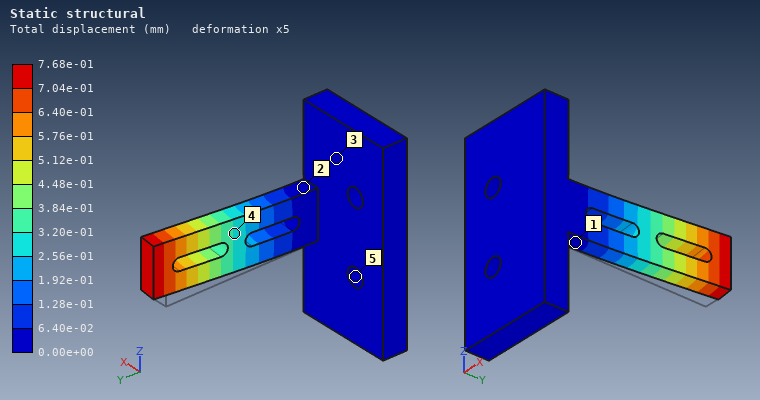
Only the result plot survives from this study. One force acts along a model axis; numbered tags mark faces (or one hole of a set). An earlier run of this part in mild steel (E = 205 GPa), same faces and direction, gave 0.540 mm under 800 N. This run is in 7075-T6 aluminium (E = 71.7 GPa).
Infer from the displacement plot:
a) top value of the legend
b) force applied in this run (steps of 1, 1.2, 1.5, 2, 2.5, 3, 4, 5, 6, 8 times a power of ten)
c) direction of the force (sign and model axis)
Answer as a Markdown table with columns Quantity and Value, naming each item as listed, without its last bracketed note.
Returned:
| Quantity | Value |
|---|---|
| top value of the legend | 7.68e-01 mm |
| force applied in this run | 400 N |
| direction of the force | +X |
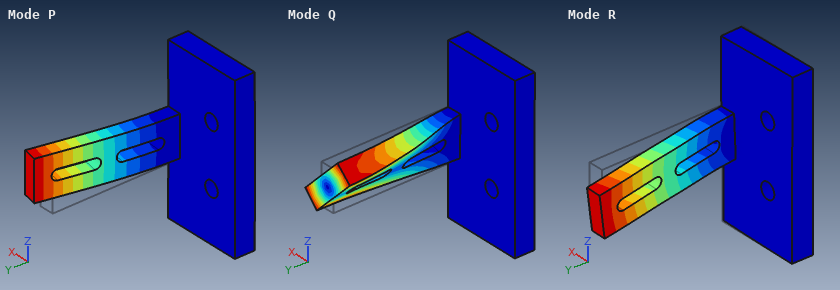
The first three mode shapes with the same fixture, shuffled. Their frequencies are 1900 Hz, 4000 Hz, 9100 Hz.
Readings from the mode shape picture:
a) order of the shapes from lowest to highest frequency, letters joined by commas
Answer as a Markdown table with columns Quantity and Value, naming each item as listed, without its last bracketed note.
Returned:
| Quantity | Value |
|---|---|
| order of the shapes from lowest to highest frequency, letters joined by commas | P, R, Q |
